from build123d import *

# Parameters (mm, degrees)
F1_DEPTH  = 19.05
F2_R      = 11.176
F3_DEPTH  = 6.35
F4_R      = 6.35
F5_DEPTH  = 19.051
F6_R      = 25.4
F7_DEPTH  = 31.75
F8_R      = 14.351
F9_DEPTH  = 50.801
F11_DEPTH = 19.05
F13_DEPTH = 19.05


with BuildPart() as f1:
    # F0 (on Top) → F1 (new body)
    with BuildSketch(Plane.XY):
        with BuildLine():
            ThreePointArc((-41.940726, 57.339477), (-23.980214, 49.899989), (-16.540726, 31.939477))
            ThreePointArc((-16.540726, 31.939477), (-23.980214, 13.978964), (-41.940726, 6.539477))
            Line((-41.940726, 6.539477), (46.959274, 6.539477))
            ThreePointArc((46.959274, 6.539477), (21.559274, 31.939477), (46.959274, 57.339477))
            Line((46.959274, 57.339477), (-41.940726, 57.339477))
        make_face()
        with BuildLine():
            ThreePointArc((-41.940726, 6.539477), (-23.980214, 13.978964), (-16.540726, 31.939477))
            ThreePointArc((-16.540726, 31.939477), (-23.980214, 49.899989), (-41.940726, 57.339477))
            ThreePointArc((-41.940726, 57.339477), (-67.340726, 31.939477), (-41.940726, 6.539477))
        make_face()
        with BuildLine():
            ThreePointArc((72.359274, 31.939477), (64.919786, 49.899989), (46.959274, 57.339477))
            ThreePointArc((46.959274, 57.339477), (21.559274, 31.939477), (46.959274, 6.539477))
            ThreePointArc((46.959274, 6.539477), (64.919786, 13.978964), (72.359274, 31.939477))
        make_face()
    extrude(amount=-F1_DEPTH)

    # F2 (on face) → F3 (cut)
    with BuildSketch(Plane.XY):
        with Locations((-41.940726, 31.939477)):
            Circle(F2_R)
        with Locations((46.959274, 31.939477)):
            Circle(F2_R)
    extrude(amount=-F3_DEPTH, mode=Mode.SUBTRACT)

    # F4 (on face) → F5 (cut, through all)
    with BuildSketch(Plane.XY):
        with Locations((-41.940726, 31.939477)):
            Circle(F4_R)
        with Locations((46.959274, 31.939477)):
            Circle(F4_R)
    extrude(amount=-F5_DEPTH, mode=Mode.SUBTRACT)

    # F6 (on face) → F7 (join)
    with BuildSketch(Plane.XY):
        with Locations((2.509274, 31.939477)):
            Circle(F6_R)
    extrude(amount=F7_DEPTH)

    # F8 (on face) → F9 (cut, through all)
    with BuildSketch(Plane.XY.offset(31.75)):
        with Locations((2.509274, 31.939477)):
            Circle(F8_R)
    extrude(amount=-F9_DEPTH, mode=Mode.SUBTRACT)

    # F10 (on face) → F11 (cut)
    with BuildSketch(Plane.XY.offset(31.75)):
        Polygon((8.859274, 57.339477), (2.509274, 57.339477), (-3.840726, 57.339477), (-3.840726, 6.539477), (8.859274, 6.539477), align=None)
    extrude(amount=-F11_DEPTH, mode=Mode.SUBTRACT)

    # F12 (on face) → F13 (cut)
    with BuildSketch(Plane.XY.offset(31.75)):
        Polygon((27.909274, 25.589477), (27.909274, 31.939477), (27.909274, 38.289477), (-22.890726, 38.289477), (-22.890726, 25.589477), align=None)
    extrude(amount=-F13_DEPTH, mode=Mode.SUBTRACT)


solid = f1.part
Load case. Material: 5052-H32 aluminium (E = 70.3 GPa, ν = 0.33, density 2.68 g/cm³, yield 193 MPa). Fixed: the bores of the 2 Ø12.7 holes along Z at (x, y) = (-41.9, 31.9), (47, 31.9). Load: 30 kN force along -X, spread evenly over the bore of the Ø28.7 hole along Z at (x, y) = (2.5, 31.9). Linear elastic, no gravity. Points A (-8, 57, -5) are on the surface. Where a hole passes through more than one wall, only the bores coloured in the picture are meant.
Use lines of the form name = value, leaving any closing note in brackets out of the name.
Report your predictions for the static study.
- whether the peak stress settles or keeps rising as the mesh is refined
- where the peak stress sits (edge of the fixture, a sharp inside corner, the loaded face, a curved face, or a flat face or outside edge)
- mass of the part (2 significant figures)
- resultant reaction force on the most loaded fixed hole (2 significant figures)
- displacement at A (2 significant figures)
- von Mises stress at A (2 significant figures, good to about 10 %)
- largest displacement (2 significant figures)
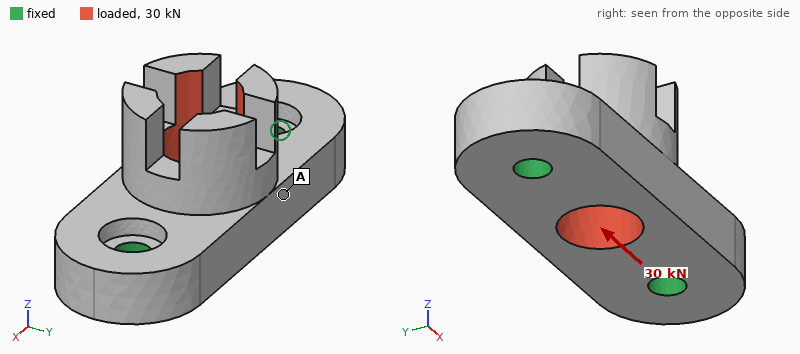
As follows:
whether the peak stress settles or keeps rising as the mesh is refined = keeps rising
where the peak stress sits = edge of the fixture
mass of the part = 370 g
resultant reaction force on the most loaded fixed hole = 16 kN
displacement at A = 11 µm
von Mises stress at A = 8.9 MPa
largest displacement = 73 µm
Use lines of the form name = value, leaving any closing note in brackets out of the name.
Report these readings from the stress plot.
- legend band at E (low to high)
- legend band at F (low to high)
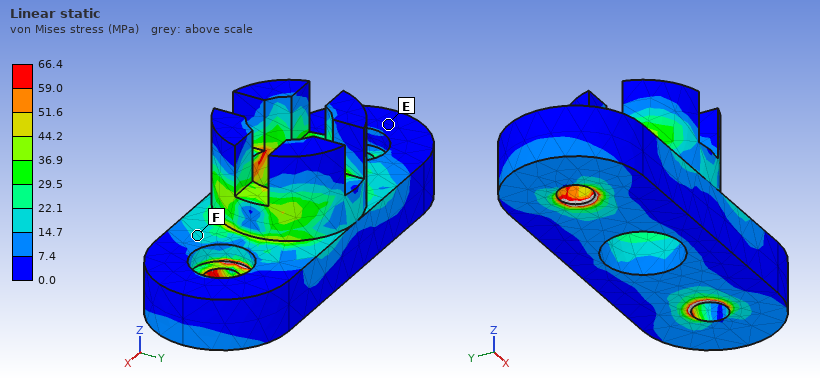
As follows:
legend band at E = 0.0 to 7.4 MPa
legend band at F = 14.7 to 22.1 MPa
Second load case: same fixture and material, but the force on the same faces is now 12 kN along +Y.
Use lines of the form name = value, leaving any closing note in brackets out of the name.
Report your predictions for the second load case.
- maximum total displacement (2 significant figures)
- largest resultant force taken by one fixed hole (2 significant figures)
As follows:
maximum total displacement = 94 µm
largest resultant force taken by one fixed hole = 6.0 kN
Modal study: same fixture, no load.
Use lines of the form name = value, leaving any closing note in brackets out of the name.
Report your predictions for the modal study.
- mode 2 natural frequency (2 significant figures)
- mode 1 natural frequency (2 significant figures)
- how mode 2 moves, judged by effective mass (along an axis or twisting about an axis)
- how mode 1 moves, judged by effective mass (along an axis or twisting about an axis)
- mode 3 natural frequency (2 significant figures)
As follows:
mode 2 natural frequency = 7500 Hz
mode 1 natural frequency = 4800 Hz
how mode 2 moves, judged by effective mass = along Z
how mode 1 moves, judged by effective mass = along Y
mode 3 natural frequency = 8500 Hz
